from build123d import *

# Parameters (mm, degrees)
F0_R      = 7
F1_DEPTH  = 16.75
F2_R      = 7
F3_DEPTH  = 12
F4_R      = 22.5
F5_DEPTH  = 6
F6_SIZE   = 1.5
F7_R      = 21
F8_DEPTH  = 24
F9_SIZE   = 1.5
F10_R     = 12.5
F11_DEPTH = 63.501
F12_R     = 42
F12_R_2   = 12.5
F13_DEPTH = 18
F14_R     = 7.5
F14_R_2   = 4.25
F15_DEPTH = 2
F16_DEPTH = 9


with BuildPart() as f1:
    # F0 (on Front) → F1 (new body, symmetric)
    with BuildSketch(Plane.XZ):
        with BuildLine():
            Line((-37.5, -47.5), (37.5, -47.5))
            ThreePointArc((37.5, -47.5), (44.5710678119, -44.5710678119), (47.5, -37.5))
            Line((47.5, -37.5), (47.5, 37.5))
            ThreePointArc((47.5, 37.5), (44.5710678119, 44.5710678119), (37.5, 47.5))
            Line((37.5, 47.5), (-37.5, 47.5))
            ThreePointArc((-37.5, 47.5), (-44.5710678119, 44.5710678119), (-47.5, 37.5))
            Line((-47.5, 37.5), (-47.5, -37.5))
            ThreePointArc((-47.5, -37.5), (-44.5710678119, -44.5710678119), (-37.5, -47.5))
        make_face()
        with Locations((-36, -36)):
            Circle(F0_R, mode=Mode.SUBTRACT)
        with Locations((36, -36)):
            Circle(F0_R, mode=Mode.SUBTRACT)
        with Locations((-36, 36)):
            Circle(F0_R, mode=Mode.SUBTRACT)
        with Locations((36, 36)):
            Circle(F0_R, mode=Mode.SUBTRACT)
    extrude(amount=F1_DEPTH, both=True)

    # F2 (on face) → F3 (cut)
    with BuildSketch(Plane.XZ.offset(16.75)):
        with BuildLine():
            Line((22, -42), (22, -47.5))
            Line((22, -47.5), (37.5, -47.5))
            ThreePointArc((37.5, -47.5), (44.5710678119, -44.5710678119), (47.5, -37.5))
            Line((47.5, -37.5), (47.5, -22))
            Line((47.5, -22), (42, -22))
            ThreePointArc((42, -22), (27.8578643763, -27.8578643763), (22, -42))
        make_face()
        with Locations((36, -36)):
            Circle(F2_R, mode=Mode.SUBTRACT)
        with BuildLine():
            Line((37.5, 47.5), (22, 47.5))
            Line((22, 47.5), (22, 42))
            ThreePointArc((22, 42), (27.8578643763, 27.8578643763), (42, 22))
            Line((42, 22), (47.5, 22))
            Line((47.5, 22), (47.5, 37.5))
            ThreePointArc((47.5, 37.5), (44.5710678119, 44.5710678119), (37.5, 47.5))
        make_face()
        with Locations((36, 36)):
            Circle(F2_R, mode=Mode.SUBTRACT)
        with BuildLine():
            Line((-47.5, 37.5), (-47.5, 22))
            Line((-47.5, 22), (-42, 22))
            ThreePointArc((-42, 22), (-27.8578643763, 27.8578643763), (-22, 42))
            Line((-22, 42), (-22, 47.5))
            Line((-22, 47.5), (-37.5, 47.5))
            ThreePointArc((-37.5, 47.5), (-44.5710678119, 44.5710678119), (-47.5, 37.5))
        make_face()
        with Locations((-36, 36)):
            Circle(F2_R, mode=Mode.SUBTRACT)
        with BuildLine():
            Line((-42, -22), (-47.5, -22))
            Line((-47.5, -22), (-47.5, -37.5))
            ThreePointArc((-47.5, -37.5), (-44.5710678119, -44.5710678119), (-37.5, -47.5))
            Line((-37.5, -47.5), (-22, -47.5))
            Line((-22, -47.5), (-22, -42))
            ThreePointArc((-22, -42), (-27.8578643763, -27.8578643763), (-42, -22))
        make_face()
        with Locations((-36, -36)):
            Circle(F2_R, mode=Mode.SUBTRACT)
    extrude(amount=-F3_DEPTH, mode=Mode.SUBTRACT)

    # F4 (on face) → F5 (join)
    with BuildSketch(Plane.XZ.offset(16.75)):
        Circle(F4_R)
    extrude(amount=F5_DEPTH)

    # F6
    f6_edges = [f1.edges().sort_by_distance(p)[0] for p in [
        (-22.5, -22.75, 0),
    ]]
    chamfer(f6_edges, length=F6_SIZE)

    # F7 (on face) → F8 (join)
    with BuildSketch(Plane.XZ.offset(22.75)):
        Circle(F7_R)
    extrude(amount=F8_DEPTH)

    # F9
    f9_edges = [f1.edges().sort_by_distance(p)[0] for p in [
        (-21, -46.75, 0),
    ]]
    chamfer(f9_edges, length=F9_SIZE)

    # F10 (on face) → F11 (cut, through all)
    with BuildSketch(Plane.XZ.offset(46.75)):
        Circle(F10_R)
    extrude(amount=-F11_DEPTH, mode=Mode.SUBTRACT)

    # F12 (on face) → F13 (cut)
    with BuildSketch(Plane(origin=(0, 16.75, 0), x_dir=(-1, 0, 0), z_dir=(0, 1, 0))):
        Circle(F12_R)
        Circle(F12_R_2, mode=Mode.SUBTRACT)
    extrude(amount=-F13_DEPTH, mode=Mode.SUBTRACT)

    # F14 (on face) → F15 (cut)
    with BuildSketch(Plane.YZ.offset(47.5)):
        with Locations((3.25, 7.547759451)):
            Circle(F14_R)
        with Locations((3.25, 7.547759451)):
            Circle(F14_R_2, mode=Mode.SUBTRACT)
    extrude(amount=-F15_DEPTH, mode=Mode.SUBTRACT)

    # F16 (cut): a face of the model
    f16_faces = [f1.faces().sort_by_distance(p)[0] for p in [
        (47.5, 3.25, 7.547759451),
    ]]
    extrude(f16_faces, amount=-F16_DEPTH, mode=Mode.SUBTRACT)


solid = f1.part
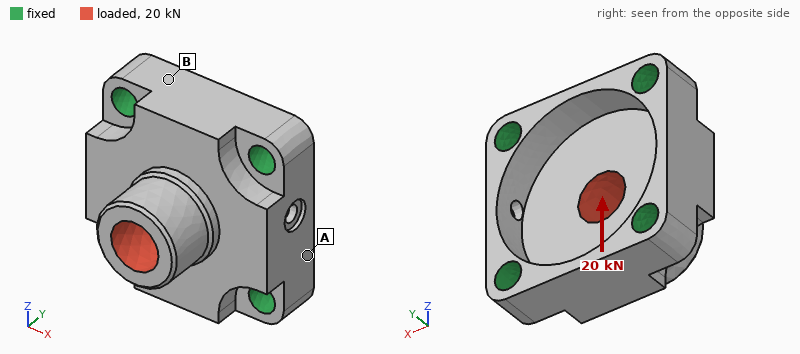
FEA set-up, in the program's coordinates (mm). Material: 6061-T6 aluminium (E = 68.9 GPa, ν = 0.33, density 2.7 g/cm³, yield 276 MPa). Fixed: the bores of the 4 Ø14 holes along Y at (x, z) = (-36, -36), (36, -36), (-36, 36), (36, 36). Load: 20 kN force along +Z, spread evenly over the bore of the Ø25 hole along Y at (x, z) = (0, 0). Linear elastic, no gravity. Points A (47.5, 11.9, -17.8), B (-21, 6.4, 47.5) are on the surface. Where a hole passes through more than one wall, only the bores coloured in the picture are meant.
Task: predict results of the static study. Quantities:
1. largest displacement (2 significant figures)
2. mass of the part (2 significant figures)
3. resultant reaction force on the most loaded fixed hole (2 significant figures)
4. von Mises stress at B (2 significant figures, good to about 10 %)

48 µm
490 g
6.5 kN
16 MPa
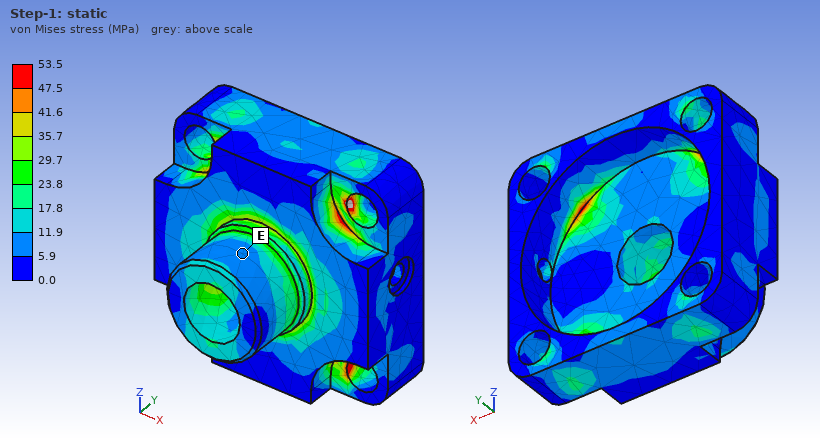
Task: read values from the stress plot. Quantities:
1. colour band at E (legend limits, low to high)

5.9 to 11.9 MPa
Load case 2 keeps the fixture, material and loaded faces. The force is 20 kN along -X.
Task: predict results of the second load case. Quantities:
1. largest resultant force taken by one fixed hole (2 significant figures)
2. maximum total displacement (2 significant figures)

6.5 kN
48 µm
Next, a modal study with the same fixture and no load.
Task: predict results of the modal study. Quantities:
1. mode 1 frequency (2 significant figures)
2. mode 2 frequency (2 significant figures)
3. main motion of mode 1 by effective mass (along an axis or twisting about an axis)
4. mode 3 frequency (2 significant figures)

9200 Hz
10 kHz
along Y
10 kHz
